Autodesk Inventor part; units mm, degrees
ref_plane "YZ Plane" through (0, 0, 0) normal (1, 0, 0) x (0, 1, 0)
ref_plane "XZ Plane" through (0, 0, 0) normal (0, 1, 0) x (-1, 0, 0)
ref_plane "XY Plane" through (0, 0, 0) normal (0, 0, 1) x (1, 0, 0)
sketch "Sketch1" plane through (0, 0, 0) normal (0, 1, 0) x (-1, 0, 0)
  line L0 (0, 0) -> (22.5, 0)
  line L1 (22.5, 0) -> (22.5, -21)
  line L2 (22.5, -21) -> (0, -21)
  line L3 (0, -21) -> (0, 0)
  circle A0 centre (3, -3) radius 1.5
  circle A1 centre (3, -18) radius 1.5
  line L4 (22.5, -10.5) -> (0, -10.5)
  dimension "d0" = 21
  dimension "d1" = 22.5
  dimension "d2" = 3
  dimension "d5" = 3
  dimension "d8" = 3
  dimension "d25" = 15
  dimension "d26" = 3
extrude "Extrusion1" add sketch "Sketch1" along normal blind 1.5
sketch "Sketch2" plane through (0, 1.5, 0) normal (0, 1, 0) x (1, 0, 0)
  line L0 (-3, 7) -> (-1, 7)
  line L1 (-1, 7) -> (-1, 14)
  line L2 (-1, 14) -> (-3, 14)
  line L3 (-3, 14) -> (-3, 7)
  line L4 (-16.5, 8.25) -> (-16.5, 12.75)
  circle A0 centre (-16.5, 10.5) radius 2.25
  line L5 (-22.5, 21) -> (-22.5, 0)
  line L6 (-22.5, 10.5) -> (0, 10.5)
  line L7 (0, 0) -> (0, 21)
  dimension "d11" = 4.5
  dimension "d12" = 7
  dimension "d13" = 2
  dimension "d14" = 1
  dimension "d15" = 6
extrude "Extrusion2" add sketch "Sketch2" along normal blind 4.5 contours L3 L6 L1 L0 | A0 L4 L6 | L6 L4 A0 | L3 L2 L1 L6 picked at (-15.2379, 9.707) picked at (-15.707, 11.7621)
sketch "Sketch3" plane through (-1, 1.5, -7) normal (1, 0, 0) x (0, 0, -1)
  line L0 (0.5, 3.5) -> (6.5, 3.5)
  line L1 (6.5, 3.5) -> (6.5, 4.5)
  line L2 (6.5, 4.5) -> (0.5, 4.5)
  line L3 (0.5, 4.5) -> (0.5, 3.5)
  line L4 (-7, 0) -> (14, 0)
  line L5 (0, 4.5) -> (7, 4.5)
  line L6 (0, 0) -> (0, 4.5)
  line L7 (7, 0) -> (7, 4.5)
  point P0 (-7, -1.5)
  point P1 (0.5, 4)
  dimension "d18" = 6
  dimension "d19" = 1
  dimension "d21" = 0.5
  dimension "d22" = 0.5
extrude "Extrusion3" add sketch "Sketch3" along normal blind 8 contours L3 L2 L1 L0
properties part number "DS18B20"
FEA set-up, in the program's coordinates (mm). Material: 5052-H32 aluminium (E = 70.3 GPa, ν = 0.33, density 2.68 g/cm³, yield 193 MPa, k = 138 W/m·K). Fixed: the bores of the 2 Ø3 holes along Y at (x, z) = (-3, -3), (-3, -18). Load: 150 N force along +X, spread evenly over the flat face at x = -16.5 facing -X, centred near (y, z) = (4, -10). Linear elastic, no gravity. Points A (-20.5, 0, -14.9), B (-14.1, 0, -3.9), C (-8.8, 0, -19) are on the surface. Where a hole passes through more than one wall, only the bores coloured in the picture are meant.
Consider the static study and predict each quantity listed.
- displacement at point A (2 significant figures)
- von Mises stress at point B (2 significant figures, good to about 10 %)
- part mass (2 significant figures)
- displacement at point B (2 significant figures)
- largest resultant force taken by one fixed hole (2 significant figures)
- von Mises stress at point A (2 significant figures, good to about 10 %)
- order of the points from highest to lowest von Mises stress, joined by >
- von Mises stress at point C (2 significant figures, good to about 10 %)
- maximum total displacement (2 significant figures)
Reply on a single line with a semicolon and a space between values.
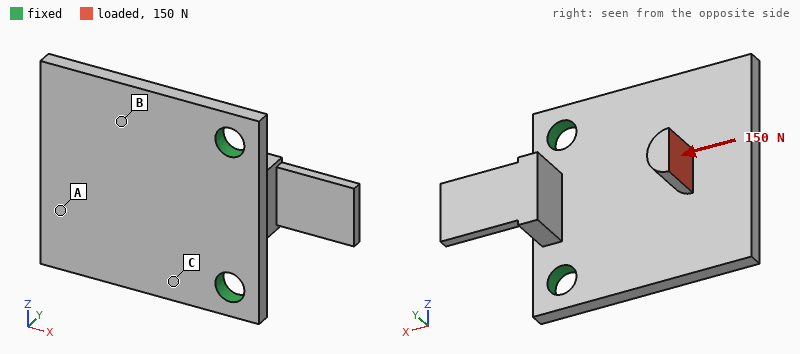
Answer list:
0.14 mm; 37 MPa; 2.2 g; 0.059 mm; 79 N; 12 MPa; C > B > A; 51 MPa; 0.17 mm
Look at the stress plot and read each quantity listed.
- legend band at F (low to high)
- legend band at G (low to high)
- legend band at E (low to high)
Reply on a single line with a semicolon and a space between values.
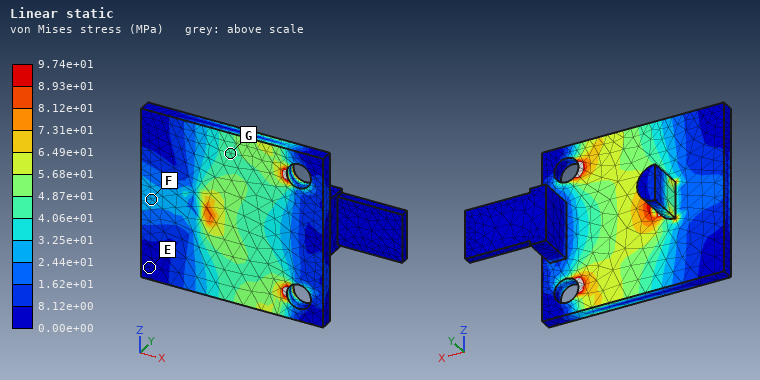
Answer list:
2.44e+01 to 3.25e+01 MPa; 4.06e+01 to 4.87e+01 MPa; 0.00e+00 to 8.12e+00 MPa
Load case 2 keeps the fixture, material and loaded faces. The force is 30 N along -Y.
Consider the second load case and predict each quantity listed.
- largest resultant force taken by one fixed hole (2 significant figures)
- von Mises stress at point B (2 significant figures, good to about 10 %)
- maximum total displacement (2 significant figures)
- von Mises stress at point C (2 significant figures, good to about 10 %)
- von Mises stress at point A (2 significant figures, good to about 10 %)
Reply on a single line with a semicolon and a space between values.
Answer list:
15 N; 10 MPa; 93 µm; 31 MPa; 6.9 MPa
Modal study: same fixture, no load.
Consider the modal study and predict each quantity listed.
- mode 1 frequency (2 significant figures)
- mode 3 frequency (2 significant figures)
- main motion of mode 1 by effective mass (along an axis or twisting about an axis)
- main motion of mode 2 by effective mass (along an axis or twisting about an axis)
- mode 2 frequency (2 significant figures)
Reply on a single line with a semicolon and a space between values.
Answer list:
3300 Hz; 9400 Hz; along Y; twisting about X; 8000 Hz
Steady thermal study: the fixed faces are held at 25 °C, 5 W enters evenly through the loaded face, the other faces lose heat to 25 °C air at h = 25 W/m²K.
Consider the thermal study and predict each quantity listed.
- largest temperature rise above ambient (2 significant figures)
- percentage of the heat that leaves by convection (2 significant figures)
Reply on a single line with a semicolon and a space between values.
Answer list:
31 K; 5.3 %
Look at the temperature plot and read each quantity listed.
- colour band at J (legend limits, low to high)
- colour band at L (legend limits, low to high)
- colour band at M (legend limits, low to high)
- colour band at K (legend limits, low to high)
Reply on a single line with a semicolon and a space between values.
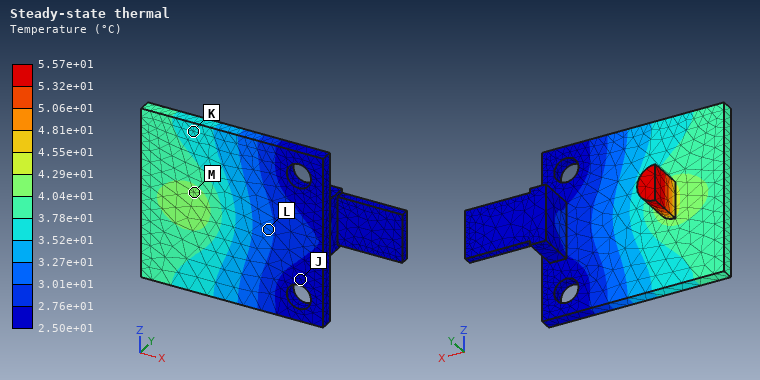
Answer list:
2.50e+01 to 2.76e+01 °C; 3.01e+01 to 3.27e+01 °C; 4.04e+01 to 4.29e+01 °C; 3.52e+01 to 3.78e+01 °C
